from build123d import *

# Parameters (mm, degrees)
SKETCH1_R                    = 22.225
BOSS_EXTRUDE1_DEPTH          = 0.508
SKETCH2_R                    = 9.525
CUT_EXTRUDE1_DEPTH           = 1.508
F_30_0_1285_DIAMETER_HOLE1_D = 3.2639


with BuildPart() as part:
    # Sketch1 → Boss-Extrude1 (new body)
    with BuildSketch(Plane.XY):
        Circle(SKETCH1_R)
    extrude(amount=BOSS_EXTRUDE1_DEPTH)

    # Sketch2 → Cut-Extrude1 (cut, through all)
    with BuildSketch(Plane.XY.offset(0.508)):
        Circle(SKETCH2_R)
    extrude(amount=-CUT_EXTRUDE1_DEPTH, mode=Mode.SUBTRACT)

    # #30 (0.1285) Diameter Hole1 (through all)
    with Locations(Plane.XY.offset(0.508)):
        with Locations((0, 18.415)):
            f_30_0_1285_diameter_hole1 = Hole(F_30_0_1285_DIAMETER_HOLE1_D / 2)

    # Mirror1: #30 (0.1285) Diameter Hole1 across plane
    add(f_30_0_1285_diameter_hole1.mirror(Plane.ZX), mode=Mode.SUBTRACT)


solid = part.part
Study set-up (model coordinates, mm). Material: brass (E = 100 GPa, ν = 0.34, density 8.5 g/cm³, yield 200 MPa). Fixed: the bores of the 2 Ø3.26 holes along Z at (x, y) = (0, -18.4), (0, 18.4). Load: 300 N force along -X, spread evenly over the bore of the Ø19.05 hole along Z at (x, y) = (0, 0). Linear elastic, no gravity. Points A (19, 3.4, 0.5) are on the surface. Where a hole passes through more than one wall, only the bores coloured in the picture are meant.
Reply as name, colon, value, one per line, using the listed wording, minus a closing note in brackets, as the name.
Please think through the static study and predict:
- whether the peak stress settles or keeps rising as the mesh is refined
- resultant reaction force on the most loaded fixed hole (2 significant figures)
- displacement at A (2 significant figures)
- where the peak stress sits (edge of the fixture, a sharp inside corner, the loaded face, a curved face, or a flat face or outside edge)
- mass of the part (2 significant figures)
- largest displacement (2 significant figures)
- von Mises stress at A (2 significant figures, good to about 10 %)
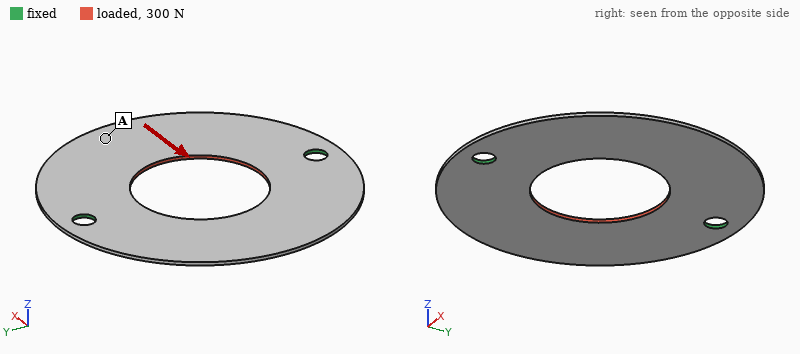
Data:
whether the peak stress settles or keeps rising as the mesh is refined: keeps rising
resultant reaction force on the most loaded fixed hole: 150 N
displacement at A: 4.1 µm
where the peak stress sits: edge of the fixture
mass of the part: 5.4 g
largest displacement: 4.9 µm
von Mises stress at A: 11 MPa
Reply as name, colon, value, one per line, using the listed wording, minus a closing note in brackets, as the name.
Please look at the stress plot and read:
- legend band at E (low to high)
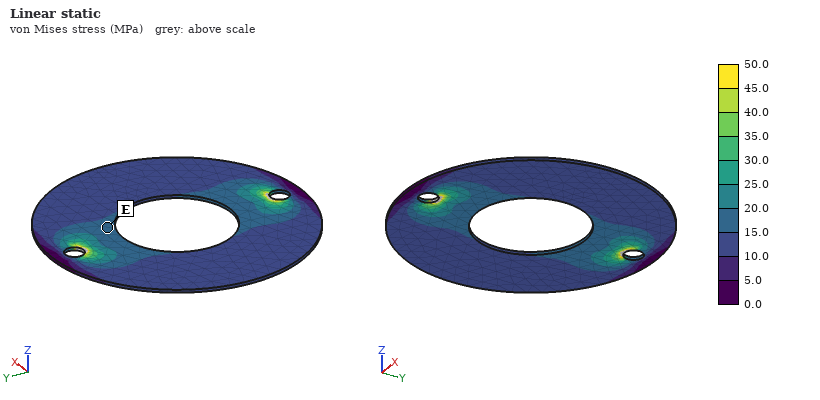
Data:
legend band at E: 15.0 to 20.0 MPa
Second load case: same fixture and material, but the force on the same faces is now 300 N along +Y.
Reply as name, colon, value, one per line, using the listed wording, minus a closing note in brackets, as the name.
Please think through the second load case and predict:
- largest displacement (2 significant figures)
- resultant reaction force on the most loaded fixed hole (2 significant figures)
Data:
largest displacement: 4.8 µm
resultant reaction force on the most loaded fixed hole: 150 N
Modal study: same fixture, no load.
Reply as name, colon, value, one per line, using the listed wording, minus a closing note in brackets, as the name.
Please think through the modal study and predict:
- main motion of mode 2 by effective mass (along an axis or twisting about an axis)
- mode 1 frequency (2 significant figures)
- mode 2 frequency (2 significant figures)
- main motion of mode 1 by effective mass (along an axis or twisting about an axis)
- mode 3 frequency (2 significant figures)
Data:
main motion of mode 2 by effective mass: along Z
mode 1 frequency: 530 Hz
mode 2 frequency: 580 Hz
main motion of mode 1 by effective mass: twisting about Y
mode 3 frequency: 1500 Hz
